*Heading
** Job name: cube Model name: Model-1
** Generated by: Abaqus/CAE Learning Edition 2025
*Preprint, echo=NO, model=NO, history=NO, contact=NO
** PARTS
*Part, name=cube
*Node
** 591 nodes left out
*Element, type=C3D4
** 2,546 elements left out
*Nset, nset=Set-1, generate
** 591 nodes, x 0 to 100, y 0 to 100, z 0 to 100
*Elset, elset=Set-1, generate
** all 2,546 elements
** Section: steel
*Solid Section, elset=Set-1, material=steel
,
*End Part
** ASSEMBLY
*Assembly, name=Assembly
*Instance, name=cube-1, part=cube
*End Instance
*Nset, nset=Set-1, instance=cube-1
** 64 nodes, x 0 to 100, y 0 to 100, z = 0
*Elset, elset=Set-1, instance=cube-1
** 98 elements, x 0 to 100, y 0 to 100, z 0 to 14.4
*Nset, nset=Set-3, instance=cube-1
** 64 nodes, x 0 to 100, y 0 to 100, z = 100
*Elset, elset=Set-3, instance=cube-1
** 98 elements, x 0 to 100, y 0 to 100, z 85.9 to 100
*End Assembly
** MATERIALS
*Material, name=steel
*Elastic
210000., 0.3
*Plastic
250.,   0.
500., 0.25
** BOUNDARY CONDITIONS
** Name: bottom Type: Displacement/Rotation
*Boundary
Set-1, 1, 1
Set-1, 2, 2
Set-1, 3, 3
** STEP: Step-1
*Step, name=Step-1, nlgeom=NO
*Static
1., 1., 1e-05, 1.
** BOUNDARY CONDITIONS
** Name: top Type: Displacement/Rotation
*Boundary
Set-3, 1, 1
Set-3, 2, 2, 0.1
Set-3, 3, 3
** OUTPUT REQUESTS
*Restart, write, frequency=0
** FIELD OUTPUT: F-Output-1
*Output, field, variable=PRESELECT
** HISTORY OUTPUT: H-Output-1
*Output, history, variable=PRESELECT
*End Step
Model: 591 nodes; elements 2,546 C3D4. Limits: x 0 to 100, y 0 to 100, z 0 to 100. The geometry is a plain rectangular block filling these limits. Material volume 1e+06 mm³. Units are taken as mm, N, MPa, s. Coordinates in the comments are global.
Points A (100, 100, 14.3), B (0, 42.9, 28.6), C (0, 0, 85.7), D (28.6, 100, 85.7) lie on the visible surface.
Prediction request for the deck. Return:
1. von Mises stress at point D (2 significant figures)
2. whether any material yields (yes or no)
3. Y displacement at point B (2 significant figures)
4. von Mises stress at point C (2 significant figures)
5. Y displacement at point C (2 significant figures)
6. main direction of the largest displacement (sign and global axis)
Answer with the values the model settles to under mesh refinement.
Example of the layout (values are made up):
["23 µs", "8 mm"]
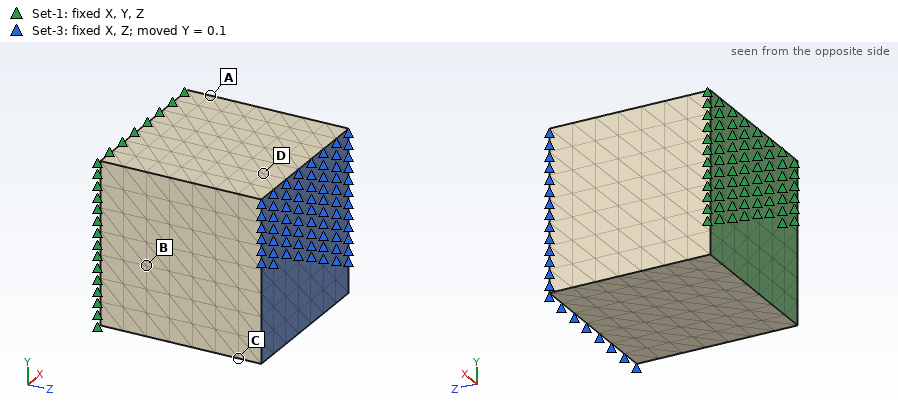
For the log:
["130 MPa", "no", "0.025 mm", "120 MPa", "0.088 mm", "+Y"]
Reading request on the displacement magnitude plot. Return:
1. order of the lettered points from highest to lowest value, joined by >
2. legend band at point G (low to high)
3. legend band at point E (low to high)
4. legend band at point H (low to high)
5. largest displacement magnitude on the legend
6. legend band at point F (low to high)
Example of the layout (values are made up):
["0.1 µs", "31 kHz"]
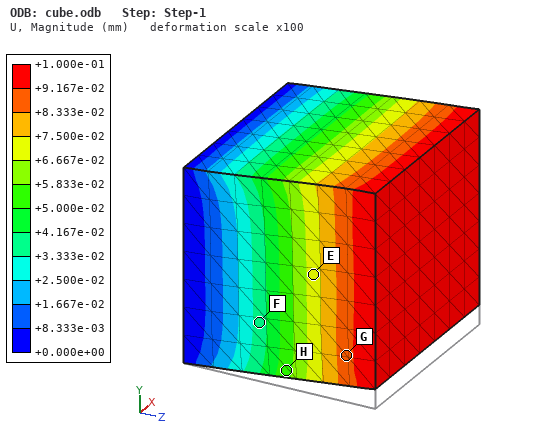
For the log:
["G > E > H > F", "+8.333e-02 to +9.167e-02 mm", "+6.667e-02 to +7.500e-02 mm", "+5.000e-02 to +5.833e-02 mm", "+1.000e-01 mm", "+3.333e-02 to +4.167e-02 mm"]
